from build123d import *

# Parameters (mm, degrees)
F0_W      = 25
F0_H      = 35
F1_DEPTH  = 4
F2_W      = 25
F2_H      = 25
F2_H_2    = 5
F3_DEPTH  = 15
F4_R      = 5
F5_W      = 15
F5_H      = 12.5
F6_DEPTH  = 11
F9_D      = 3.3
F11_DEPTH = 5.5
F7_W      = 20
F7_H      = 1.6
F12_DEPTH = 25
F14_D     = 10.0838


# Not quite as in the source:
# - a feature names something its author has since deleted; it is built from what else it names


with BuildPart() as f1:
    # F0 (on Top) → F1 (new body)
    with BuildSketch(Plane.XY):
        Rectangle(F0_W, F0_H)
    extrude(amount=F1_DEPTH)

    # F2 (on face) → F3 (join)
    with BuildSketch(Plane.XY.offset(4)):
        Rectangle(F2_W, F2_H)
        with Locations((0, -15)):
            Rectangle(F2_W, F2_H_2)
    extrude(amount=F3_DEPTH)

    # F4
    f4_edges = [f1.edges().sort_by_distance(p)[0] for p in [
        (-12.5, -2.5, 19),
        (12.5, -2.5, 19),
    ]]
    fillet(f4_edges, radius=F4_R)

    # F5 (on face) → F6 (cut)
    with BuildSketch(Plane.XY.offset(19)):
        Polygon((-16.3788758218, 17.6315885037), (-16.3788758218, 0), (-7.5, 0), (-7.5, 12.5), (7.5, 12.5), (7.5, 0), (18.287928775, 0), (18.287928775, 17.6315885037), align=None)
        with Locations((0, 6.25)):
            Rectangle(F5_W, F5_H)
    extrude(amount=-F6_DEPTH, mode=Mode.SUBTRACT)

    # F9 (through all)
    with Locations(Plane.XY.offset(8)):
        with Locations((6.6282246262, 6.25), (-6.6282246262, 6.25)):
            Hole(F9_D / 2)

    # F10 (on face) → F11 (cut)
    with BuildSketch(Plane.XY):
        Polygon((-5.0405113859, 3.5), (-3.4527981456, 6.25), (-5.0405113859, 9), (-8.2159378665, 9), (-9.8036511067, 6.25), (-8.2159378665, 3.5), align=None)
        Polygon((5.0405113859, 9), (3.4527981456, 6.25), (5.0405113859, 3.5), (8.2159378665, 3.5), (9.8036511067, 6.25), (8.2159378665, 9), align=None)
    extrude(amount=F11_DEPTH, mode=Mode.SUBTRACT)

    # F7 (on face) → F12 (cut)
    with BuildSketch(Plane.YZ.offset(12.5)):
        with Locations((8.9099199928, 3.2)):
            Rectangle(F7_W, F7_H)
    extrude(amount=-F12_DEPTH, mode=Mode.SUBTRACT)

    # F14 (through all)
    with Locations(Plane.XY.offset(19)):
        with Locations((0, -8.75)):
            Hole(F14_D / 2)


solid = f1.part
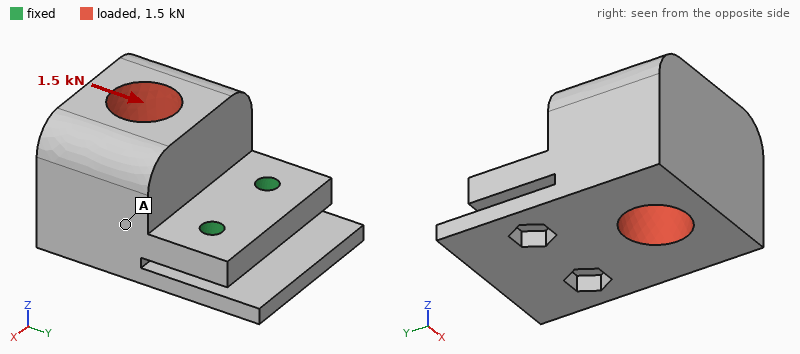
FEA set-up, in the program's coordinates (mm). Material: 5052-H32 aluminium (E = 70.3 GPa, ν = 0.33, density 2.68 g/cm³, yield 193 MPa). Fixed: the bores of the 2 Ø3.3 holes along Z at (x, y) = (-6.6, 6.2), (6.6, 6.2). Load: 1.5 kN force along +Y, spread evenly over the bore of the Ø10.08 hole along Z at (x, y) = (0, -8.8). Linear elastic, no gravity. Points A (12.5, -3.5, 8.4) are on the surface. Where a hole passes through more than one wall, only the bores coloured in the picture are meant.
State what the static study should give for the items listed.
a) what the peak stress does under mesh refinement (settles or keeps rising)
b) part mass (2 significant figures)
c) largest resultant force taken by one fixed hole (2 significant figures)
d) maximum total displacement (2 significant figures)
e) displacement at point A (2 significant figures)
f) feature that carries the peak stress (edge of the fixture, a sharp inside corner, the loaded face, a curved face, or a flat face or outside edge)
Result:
keeps rising
23 g
760 N
0.13 mm
0.037 mm
edge of the fixture
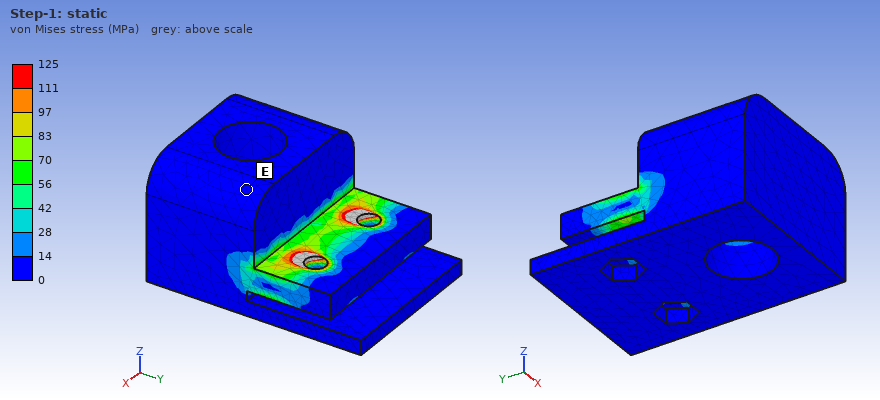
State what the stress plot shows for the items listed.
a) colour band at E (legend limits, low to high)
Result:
0 to 14 MPa
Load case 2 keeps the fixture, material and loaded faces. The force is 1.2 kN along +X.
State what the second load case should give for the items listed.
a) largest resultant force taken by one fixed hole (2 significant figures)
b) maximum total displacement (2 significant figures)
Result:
1.3 kN
34 µm
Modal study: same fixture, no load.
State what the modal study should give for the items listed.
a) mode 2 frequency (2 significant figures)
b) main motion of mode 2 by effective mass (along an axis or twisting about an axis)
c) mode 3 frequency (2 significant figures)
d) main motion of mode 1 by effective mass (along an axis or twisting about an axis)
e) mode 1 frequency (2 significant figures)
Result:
4600 Hz
along Z
7300 Hz
along Z
2300 Hz
